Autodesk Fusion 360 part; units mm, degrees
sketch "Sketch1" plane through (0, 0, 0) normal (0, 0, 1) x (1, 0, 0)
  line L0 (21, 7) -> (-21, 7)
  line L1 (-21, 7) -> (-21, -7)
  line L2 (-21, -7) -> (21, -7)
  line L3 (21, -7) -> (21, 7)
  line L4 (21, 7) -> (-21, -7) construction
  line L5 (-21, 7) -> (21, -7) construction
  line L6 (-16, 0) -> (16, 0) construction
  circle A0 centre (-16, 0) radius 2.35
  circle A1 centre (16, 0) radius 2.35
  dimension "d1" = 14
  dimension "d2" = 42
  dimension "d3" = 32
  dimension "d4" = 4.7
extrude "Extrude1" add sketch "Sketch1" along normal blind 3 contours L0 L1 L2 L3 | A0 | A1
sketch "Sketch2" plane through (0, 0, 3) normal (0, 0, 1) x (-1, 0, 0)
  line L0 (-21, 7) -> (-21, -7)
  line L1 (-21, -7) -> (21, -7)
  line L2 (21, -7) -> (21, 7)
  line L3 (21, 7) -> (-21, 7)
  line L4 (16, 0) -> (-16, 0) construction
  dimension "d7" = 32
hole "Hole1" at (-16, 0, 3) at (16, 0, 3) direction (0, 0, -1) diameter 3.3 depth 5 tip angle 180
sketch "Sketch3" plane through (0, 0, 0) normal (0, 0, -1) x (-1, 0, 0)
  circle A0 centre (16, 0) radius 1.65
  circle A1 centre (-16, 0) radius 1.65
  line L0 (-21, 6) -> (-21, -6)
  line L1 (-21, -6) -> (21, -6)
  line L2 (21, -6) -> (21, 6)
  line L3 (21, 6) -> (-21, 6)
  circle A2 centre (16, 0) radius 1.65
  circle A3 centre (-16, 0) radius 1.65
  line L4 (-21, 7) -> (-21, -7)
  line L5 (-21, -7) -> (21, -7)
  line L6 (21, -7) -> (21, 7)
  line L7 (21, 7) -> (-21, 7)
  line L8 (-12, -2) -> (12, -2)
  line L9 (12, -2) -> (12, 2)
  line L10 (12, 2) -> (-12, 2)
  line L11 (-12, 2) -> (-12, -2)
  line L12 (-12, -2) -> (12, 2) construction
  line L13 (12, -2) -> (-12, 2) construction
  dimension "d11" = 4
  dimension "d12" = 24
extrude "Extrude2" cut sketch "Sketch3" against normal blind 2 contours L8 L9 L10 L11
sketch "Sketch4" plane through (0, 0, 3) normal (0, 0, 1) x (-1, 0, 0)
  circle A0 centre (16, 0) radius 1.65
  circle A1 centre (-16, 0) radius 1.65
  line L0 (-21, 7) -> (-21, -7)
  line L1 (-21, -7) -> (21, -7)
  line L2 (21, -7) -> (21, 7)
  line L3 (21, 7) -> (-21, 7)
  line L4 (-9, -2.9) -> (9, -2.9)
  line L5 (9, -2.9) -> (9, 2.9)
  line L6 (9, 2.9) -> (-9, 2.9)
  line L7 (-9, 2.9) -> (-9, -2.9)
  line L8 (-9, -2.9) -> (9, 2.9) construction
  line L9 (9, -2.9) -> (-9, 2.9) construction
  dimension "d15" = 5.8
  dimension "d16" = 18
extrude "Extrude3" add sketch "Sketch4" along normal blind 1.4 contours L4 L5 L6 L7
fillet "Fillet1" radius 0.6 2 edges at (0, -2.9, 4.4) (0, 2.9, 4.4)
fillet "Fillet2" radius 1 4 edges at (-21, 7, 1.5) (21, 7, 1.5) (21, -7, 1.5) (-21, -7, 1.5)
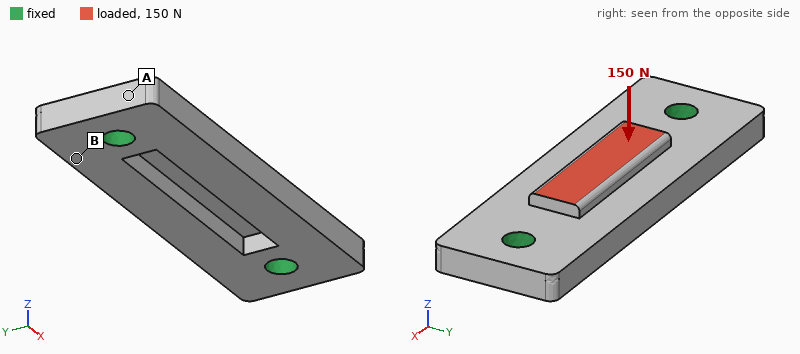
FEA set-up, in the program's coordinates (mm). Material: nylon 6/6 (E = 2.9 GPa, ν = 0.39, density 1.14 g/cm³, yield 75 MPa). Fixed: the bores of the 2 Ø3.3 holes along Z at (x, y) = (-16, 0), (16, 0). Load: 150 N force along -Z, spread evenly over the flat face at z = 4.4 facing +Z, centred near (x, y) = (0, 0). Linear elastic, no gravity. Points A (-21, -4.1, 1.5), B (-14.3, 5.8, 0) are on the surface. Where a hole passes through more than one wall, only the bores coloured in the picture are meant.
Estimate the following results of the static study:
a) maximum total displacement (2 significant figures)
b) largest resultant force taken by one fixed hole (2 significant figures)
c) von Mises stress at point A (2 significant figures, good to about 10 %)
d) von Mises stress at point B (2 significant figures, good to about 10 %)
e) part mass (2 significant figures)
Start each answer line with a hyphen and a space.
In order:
- 0.20 mm
- 82 N
- 2.5 MPa
- 9.0 MPa
- 1.9 g
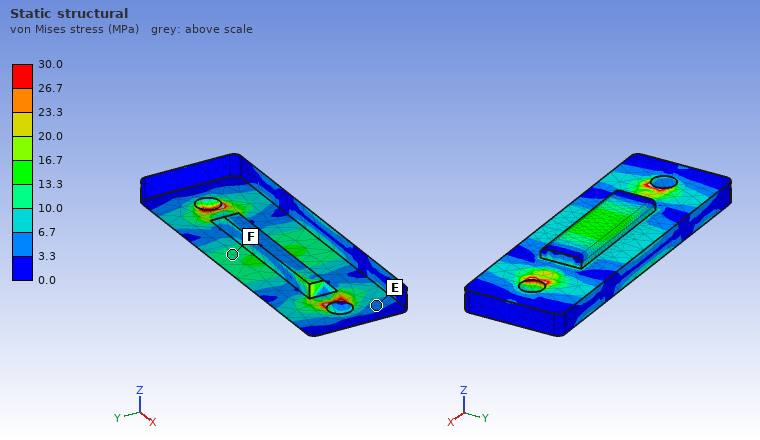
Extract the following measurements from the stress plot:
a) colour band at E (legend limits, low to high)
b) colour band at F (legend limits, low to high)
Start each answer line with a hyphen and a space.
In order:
- 3.3 to 6.7 MPa
- 10.0 to 13.3 MPa
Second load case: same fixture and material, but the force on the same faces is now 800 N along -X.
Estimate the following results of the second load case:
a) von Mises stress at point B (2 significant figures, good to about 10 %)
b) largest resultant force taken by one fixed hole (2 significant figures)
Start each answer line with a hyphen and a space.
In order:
- 6.8 MPa
- 410 N
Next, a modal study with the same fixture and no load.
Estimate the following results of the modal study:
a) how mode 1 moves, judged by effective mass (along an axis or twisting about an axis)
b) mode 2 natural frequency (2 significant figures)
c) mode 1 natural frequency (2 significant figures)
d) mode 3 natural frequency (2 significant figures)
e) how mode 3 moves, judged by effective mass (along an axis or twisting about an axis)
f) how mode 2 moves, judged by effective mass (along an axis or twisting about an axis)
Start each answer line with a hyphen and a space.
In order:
- along Z
- 5900 Hz
- 4800 Hz
- 8700 Hz
- along Y
- twisting about X
